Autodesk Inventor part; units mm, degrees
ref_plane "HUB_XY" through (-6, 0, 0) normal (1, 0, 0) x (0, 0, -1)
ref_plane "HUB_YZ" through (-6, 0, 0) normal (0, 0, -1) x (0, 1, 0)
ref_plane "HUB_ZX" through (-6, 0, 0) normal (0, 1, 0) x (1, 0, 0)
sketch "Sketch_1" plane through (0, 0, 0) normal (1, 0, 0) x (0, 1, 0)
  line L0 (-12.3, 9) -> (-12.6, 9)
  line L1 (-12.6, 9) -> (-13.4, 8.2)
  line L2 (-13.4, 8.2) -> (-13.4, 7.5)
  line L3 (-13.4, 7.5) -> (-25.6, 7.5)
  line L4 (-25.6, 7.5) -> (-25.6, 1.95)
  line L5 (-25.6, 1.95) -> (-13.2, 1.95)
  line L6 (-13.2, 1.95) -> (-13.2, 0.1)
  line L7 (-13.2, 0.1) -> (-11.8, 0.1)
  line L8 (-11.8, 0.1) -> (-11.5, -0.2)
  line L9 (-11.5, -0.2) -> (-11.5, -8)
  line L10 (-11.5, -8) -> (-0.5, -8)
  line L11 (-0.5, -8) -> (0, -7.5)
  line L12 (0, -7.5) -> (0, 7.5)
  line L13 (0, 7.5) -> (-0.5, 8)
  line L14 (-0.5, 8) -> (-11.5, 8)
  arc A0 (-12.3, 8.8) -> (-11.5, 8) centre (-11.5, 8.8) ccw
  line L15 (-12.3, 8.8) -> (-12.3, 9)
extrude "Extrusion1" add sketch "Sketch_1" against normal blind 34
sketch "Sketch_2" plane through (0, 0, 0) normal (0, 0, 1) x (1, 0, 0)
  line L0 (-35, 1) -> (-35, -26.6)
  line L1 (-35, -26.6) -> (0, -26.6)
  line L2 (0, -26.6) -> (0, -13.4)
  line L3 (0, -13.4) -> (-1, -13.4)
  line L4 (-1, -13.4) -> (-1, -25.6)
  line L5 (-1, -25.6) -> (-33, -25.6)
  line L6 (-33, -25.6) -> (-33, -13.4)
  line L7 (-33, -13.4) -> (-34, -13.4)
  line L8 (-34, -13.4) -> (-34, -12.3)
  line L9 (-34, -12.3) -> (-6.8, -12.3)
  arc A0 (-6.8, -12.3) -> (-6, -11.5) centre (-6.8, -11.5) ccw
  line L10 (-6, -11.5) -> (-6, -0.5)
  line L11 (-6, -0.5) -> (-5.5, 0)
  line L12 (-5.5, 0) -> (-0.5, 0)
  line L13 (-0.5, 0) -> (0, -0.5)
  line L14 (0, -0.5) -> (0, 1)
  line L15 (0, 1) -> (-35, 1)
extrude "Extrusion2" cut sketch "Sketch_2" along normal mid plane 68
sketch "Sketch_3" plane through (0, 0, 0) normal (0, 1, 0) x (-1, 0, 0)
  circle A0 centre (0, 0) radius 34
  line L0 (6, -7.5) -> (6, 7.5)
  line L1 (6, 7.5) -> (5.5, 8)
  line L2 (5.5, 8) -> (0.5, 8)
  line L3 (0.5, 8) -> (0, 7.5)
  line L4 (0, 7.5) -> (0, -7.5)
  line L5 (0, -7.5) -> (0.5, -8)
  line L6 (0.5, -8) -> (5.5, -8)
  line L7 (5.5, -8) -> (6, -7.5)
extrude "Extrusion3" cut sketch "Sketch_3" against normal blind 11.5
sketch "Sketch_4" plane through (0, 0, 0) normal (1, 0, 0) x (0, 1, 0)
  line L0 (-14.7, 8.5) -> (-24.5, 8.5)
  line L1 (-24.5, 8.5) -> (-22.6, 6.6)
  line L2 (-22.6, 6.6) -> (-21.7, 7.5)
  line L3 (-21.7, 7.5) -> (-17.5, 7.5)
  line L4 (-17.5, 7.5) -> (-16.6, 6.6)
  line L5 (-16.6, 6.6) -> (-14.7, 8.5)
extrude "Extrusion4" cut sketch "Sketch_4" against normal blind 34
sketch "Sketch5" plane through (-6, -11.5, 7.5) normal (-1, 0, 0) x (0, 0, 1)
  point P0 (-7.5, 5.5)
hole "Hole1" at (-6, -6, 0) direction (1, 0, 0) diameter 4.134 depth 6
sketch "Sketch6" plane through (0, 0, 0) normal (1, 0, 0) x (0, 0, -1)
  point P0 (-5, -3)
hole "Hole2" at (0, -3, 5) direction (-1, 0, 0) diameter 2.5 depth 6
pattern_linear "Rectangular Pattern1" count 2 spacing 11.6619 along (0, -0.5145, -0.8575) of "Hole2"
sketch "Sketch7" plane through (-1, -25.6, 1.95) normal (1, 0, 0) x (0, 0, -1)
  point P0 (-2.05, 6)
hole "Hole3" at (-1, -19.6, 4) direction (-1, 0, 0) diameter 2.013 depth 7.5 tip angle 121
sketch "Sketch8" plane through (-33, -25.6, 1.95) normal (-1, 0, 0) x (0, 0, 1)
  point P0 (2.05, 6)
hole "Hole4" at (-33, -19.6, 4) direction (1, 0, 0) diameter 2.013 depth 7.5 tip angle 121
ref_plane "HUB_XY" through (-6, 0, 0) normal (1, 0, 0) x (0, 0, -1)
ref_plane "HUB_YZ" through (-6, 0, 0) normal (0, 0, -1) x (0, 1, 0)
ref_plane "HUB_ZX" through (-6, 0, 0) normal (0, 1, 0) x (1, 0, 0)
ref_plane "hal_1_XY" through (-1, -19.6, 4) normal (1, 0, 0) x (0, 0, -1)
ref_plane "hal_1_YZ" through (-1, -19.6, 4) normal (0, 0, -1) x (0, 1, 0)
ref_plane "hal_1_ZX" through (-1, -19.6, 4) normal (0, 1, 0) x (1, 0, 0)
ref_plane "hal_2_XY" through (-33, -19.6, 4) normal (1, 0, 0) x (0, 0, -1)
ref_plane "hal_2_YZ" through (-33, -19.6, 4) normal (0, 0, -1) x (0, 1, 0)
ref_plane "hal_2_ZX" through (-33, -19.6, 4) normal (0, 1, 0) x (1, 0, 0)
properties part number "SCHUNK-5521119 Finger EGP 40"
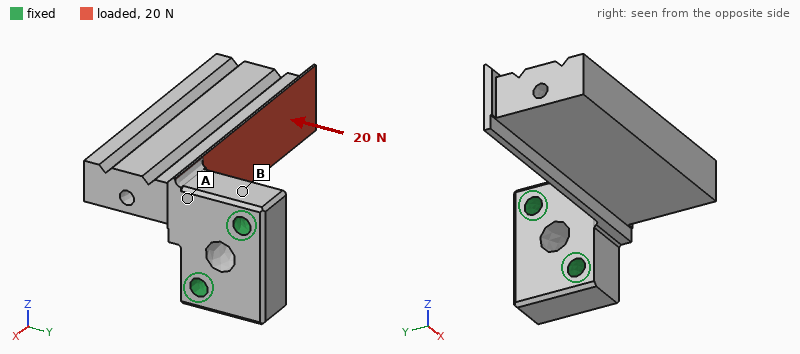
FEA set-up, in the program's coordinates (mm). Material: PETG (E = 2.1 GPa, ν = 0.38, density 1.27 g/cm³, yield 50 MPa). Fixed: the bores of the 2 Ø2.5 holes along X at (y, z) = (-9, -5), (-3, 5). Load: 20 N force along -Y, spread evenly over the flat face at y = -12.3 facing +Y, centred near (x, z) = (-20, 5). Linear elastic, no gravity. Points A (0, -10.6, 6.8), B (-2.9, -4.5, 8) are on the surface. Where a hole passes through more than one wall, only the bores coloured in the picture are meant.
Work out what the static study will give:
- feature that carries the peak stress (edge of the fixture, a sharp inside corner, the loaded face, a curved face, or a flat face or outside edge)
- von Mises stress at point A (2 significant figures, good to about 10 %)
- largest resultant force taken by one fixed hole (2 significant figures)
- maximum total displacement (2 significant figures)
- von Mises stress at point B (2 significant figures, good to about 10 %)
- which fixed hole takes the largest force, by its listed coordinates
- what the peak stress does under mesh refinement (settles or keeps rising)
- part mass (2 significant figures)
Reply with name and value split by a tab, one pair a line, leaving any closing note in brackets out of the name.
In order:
feature that carries the peak stress	a sharp inside corner
von Mises stress at point A	6.1 MPa
largest resultant force taken by one fixed hole	22 N
maximum total displacement	0.55 mm
von Mises stress at point B	2.0 MPa
which fixed hole takes the largest force, by its listed coordinates	(-3, 5)
what the peak stress does under mesh refinement	keeps rising
part mass	4.3 g
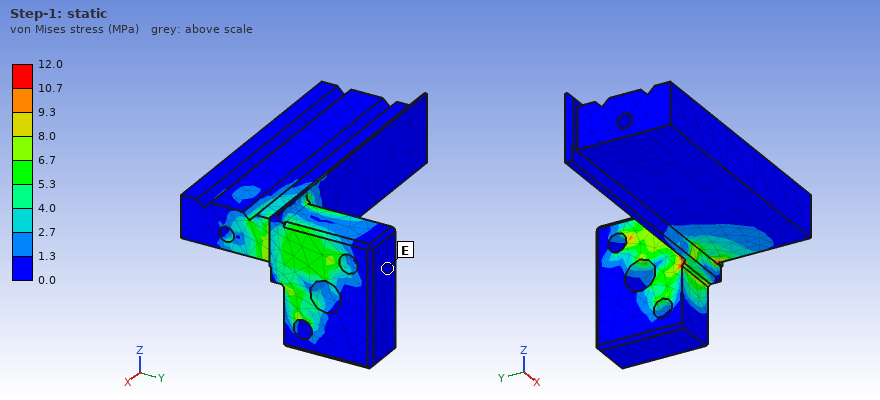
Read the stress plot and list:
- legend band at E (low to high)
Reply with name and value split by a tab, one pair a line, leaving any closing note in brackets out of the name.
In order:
legend band at E	0.0 to 1.3 MPa
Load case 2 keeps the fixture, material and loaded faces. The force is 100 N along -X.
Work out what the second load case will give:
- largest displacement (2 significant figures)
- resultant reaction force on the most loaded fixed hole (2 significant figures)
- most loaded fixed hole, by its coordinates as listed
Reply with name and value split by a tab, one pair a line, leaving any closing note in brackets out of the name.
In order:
largest displacement	0.29 mm
resultant reaction force on the most loaded fixed hole	58 N
most loaded fixed hole, by its coordinates as listed	(-3, 5)
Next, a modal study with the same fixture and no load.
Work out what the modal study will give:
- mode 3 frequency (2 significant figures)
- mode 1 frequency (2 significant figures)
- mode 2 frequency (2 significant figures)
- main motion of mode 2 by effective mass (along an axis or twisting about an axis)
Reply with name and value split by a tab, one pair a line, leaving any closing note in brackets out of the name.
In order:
mode 3 frequency	2400 Hz
mode 1 frequency	700 Hz
mode 2 frequency	800 Hz
main motion of mode 2 by effective mass	along Z
